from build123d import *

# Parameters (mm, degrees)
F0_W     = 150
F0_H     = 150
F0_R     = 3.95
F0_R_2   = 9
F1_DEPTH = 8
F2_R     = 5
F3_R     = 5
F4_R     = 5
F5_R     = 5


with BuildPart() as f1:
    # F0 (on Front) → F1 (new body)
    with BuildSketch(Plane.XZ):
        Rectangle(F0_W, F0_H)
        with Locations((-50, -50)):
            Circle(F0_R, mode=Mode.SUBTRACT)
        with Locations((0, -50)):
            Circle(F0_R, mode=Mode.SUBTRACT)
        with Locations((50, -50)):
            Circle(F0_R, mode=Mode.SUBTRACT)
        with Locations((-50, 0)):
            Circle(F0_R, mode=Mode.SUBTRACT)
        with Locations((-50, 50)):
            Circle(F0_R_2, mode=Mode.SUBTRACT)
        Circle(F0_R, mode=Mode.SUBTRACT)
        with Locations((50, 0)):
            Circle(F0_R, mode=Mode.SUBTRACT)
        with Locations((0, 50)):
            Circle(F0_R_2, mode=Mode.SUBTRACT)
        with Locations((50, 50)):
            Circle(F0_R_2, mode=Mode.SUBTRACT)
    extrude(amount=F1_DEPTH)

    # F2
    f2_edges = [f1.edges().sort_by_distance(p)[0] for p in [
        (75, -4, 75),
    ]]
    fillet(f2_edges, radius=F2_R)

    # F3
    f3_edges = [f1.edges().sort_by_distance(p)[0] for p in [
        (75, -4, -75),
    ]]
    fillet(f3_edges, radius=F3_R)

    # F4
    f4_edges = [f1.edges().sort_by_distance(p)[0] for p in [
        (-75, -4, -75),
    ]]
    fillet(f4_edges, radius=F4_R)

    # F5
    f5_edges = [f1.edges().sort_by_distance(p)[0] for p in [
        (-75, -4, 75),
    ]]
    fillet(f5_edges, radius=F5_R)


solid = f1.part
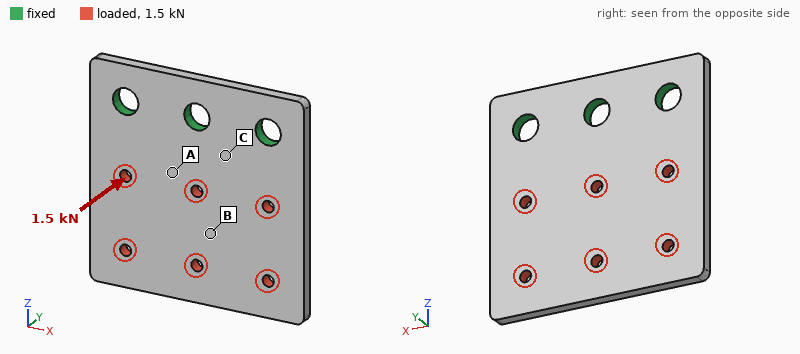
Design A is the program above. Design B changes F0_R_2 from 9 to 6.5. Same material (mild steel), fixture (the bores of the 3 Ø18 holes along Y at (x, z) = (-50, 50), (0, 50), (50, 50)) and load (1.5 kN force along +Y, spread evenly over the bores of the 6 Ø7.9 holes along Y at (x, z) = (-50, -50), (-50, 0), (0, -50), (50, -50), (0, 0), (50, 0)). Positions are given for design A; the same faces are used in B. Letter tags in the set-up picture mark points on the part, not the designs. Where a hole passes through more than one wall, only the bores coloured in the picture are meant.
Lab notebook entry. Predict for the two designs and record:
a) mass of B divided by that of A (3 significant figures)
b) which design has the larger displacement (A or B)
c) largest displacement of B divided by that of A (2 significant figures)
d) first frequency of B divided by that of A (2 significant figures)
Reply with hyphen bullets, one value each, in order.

- 1.02
- B
- 1.1
- 0.95
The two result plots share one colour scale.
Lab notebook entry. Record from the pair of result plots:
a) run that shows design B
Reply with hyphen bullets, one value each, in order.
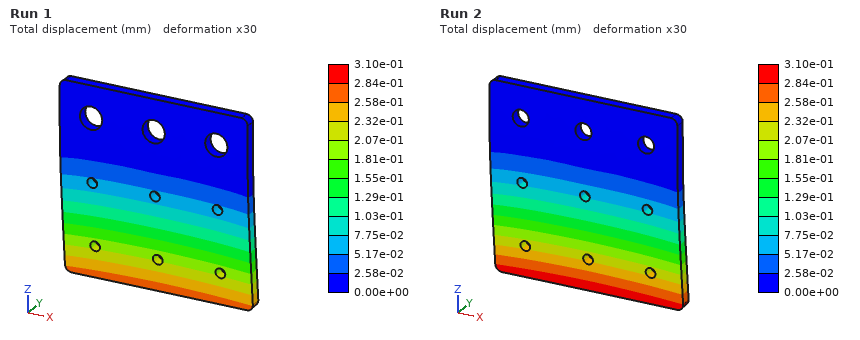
- Run 2
